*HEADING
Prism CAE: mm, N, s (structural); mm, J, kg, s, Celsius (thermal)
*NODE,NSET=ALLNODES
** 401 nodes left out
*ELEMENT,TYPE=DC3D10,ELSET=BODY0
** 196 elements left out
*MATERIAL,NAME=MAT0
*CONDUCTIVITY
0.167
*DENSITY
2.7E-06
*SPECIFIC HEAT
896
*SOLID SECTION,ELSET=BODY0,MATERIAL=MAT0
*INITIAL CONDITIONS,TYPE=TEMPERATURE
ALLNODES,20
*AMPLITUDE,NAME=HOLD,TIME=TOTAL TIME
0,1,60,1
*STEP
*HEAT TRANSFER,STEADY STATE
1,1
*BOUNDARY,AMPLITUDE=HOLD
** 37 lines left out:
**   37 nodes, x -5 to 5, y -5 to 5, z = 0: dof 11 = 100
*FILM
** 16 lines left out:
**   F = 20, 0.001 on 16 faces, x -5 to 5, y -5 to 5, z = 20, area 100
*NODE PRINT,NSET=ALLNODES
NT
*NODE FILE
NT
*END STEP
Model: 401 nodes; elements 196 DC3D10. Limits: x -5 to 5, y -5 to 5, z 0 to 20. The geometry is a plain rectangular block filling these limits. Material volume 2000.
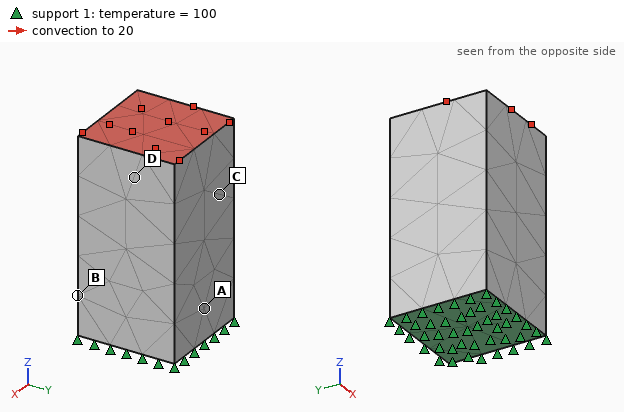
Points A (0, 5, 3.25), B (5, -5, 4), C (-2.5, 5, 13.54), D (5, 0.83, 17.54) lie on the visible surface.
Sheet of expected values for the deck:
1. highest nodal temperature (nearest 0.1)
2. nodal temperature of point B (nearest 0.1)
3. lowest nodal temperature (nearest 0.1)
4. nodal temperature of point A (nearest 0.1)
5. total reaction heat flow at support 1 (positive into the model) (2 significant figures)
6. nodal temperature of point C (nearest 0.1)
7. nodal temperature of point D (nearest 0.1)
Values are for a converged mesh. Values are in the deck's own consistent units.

100.0
98.3
91.4
98.6
7.1
94.2
92.5
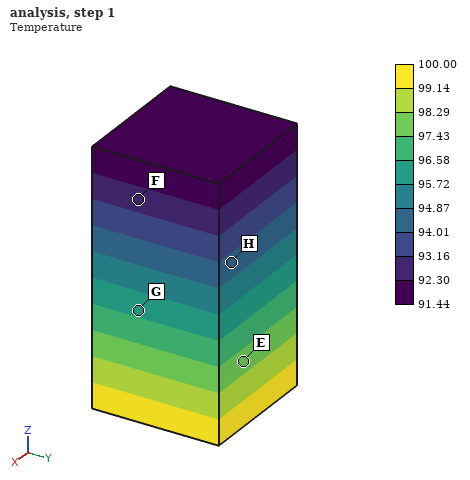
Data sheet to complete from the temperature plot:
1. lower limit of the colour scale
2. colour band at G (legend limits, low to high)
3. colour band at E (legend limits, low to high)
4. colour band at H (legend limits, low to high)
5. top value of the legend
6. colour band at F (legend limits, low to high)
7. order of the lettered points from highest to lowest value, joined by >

91.44
95.72 to 96.58
97.43 to 98.29
94.01 to 94.87
100.00
92.30 to 93.16
E > G > H > F
